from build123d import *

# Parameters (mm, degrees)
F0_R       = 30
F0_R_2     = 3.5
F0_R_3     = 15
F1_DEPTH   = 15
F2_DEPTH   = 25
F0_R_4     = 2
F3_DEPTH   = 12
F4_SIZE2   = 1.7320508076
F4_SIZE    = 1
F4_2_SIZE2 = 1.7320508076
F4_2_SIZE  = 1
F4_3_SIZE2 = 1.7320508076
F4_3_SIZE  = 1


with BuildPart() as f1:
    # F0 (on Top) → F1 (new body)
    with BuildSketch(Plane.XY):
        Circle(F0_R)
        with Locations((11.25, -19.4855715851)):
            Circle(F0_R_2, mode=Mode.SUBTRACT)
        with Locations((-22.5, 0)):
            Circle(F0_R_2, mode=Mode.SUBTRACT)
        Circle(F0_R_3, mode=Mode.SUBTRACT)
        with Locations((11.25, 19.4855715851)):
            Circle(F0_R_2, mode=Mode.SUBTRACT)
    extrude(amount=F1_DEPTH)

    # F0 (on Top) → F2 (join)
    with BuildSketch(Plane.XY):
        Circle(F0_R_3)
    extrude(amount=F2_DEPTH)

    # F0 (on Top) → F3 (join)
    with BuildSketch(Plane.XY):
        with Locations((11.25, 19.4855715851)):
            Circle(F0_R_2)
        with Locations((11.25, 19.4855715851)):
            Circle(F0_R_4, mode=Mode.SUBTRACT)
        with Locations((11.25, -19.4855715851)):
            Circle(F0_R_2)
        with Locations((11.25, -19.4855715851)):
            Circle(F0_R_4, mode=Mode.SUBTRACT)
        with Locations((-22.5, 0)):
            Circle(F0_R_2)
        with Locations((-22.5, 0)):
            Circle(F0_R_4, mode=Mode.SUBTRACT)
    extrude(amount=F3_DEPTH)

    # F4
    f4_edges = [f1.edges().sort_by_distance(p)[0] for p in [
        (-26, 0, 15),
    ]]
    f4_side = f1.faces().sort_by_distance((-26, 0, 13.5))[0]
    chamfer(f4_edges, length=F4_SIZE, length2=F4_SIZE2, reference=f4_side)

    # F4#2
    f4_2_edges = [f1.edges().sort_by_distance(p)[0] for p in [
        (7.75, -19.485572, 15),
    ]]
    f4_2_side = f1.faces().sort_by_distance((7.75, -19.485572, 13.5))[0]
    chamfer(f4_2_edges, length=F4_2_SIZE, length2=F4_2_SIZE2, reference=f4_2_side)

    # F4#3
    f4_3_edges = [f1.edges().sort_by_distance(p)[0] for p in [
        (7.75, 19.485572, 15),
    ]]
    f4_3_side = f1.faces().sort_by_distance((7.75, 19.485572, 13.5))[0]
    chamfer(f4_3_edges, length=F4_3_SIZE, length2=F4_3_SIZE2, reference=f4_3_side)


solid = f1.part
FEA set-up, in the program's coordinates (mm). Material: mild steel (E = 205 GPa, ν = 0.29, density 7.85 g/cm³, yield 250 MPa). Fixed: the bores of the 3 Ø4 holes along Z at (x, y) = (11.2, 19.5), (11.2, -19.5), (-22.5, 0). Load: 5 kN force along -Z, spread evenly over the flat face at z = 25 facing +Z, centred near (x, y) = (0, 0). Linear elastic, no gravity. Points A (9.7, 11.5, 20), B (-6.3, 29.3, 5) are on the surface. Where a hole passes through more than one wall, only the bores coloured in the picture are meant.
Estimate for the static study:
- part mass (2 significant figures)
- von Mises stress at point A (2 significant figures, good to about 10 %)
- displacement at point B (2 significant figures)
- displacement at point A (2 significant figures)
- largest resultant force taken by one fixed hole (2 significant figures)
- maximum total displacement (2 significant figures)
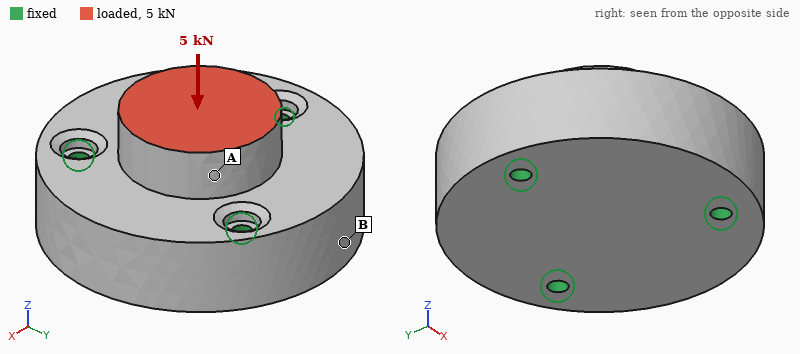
380 g
9.6 MPa
0.75 µm
1.5 µm
1.7 kN
1.7 µm
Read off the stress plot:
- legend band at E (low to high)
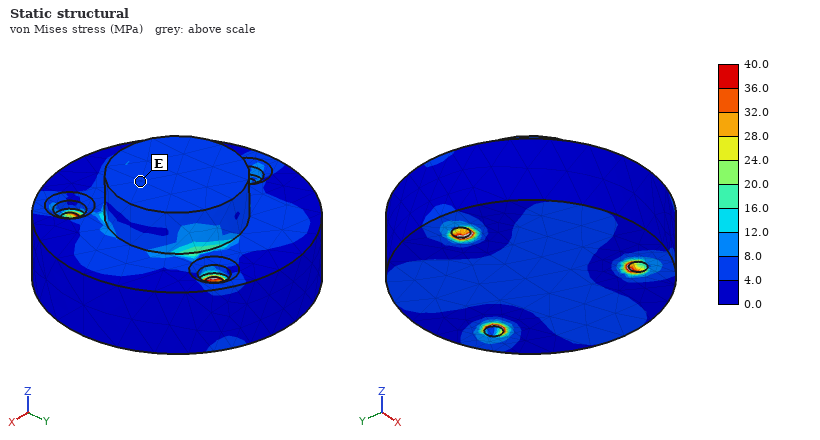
4.0 to 8.0 MPa
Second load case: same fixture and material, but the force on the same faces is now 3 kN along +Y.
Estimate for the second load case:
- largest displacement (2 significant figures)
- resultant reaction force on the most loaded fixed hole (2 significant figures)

2.7 µm
1.7 kN
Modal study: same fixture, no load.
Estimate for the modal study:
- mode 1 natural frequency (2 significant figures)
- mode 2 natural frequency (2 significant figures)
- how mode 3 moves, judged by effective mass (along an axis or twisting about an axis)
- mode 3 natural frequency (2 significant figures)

18 kHz
18 kHz
along Z
19 kHz
